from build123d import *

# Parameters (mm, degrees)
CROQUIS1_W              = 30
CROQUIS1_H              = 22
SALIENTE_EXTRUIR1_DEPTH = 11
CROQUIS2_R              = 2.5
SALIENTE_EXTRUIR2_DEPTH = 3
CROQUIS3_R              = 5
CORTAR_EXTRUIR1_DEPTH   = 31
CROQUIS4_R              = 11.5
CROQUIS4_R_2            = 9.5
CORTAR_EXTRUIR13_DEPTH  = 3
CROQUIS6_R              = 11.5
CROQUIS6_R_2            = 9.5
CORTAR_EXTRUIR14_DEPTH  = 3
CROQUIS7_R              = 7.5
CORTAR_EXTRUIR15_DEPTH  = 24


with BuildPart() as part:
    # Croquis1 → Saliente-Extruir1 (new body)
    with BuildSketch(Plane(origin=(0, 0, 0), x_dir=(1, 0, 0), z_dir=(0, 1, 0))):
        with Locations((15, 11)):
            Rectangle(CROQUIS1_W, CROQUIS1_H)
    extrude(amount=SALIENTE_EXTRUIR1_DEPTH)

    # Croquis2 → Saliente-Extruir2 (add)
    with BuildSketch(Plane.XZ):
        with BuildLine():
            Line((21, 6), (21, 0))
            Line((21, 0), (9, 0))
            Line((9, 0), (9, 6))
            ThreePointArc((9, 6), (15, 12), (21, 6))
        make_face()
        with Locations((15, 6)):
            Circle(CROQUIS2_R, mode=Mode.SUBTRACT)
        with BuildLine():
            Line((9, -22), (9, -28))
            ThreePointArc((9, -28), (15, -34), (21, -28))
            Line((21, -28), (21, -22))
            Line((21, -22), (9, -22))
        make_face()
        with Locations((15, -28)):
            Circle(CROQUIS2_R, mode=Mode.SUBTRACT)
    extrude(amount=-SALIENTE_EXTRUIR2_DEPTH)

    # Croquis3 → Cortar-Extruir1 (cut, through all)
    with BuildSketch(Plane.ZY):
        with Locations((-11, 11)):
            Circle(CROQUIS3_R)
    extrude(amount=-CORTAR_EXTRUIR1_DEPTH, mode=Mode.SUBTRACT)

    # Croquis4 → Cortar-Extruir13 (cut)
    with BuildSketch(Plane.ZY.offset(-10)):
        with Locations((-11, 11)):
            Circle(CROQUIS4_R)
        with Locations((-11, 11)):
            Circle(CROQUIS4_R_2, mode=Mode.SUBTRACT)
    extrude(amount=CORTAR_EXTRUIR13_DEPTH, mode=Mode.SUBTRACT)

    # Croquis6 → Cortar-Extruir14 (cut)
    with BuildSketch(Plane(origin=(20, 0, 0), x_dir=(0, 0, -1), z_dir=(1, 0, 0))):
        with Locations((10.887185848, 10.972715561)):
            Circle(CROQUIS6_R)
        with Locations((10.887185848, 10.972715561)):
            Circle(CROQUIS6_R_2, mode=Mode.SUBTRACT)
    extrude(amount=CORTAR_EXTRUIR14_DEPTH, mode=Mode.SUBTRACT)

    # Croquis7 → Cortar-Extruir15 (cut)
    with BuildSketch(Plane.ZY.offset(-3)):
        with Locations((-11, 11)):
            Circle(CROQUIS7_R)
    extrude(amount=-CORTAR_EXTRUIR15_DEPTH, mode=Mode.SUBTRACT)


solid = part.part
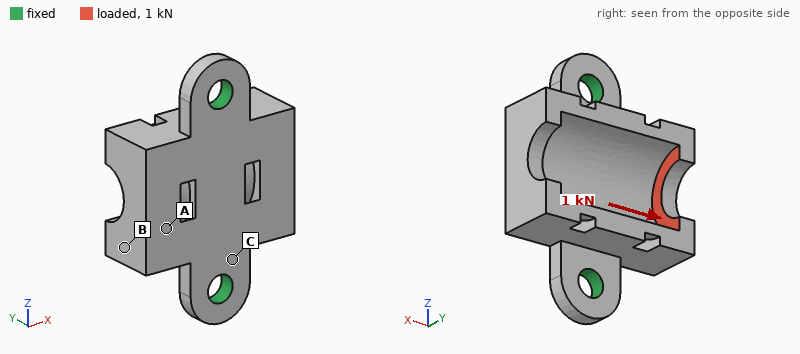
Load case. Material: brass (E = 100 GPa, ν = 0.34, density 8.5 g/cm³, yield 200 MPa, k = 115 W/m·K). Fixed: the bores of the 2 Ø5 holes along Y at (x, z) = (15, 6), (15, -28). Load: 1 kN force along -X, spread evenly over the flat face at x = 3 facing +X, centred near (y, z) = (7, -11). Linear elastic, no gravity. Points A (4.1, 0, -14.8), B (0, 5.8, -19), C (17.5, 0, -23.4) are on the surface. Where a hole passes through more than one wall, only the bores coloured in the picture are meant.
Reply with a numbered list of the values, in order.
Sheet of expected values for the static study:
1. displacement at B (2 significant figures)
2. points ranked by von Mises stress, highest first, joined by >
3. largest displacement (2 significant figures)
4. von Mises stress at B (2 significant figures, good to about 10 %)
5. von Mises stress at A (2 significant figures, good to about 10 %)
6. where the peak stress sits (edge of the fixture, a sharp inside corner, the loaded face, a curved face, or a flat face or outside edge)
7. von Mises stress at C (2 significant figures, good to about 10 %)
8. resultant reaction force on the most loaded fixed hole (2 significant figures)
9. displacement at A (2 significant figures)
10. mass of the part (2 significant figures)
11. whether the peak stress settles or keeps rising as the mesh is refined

1. 48 µm
2. C > B > A
3. 59 µm
4. 25 MPa
5. 12 MPa
6. edge of the fixture
7. 40 MPa
8. 500 N
9. 32 µm
10. 44 g
11. keeps rising
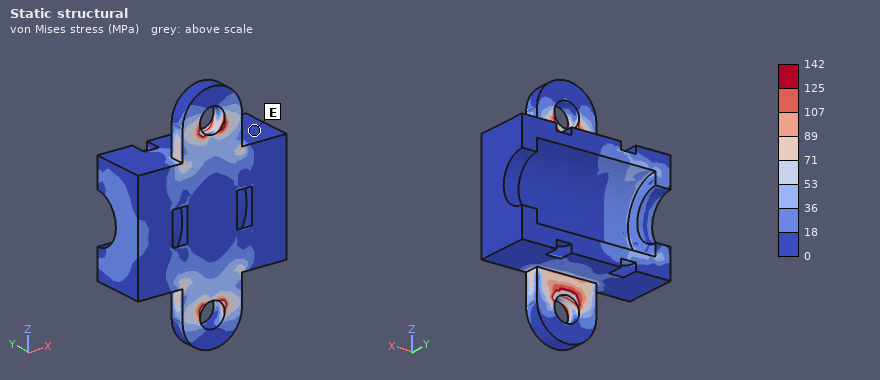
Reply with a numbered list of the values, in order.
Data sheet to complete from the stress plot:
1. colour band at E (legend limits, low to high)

1. 0 to 18 MPa
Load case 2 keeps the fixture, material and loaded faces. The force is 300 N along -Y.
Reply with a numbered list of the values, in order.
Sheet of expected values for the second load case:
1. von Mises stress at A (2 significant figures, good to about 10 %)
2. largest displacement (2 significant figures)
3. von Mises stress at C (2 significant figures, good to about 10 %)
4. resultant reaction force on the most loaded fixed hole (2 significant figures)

1. 13 MPa
2. 38 µm
3. 43 MPa
4. 180 N
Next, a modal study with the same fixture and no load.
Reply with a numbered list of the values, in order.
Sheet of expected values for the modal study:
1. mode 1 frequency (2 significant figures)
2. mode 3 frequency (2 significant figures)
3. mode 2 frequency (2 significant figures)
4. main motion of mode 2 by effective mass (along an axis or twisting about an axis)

1. 3600 Hz
2. 12 kHz
3. 7300 Hz
4. along Y
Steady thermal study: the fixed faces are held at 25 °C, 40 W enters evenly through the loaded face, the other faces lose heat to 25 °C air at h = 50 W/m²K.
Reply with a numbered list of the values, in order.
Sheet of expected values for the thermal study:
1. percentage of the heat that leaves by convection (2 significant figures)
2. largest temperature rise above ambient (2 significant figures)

1. 14 %
2. 76 K
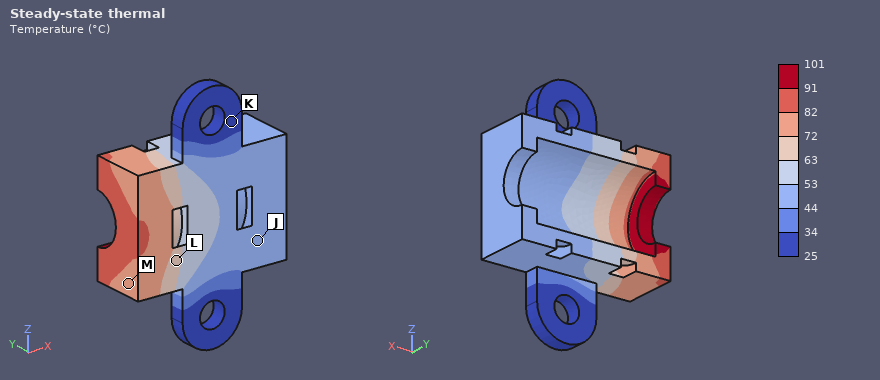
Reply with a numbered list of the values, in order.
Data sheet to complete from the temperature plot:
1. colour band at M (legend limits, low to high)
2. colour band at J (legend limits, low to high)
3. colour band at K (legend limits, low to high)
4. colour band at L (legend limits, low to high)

1. 72 to 82 °C
2. 44 to 53 °C
3. 25 to 34 °C
4. 63 to 72 °C
